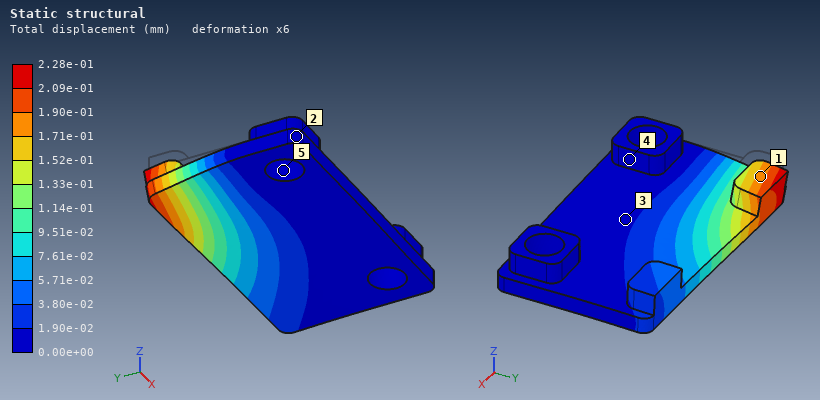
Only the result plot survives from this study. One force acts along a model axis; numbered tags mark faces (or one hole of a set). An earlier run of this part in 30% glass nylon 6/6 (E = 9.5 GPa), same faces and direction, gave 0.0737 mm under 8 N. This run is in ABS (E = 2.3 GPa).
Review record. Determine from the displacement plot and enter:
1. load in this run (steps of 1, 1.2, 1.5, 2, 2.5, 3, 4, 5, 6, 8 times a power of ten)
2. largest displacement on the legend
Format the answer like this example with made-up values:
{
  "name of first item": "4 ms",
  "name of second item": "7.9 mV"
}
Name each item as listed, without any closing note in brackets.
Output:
{
  "load in this run": "6 N",
  "largest displacement on the legend": "2.28e-01 mm"
}
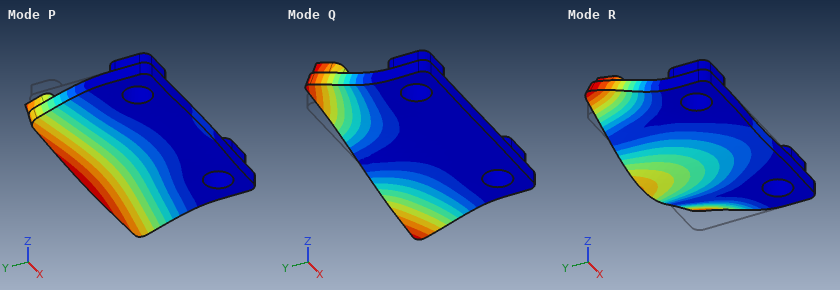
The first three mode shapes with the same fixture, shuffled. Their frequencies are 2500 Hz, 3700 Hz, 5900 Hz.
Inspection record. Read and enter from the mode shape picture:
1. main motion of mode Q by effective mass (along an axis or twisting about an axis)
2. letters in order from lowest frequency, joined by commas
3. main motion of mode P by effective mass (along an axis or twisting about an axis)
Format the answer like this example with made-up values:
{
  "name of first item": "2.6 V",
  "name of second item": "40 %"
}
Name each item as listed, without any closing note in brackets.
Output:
{
  "main motion of mode Q by effective mass": "twisting about Y",
  "letters in order from lowest frequency, joined by commas": "P, Q, R",
  "main motion of mode P by effective mass": "along Z"
}
